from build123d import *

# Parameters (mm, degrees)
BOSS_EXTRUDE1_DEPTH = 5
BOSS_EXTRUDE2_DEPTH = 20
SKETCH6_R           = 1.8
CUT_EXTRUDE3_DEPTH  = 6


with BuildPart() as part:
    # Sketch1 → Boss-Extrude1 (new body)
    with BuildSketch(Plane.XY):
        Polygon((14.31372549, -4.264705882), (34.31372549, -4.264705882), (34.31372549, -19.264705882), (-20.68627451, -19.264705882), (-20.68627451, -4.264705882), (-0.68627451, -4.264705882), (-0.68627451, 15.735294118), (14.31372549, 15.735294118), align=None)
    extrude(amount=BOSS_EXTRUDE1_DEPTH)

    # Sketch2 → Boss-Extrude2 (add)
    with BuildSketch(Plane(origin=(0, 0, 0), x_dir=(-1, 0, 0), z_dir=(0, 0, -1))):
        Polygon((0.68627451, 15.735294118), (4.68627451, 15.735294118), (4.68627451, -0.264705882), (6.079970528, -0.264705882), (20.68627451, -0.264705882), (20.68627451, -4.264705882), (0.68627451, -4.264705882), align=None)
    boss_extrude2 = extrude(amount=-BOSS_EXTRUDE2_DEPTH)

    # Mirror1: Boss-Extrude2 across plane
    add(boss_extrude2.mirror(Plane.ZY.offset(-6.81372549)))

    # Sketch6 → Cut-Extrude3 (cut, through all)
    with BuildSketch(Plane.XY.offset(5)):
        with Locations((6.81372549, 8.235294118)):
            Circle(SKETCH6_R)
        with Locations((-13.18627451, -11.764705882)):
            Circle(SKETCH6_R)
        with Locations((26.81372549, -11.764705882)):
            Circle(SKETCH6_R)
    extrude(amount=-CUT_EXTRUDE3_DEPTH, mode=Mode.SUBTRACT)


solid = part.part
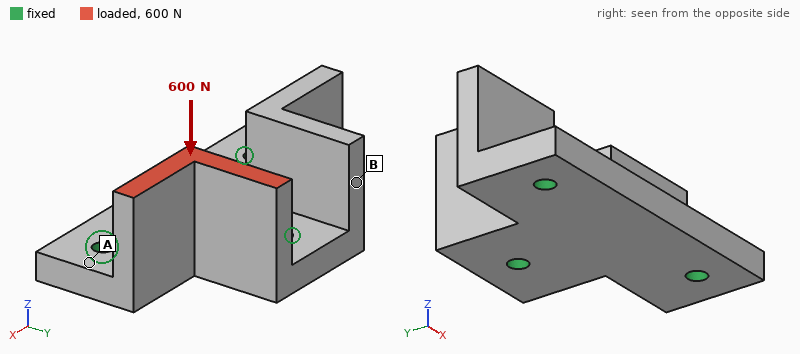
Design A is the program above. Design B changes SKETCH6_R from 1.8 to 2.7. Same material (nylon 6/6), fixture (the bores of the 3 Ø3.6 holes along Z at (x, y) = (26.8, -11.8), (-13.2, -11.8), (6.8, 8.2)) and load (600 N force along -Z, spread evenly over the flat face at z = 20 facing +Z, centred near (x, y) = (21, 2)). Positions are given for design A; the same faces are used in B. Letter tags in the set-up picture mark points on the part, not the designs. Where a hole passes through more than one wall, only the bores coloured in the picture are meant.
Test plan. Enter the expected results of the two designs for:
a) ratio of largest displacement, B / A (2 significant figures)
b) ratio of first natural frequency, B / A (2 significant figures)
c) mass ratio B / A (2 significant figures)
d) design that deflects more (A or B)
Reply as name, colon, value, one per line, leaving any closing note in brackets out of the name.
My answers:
ratio of largest displacement, B / A: 0.74
ratio of first natural frequency, B / A: 1.1
mass ratio B / A: 0.98
design that deflects more: A
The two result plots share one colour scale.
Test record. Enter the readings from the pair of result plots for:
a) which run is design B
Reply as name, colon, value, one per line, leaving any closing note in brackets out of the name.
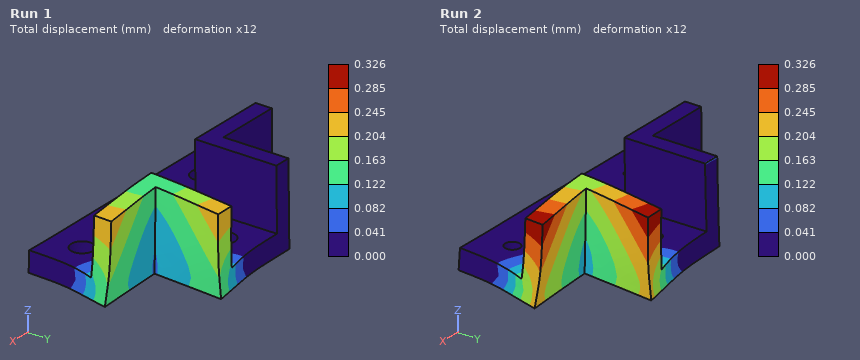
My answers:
which run is design B: Run 1
